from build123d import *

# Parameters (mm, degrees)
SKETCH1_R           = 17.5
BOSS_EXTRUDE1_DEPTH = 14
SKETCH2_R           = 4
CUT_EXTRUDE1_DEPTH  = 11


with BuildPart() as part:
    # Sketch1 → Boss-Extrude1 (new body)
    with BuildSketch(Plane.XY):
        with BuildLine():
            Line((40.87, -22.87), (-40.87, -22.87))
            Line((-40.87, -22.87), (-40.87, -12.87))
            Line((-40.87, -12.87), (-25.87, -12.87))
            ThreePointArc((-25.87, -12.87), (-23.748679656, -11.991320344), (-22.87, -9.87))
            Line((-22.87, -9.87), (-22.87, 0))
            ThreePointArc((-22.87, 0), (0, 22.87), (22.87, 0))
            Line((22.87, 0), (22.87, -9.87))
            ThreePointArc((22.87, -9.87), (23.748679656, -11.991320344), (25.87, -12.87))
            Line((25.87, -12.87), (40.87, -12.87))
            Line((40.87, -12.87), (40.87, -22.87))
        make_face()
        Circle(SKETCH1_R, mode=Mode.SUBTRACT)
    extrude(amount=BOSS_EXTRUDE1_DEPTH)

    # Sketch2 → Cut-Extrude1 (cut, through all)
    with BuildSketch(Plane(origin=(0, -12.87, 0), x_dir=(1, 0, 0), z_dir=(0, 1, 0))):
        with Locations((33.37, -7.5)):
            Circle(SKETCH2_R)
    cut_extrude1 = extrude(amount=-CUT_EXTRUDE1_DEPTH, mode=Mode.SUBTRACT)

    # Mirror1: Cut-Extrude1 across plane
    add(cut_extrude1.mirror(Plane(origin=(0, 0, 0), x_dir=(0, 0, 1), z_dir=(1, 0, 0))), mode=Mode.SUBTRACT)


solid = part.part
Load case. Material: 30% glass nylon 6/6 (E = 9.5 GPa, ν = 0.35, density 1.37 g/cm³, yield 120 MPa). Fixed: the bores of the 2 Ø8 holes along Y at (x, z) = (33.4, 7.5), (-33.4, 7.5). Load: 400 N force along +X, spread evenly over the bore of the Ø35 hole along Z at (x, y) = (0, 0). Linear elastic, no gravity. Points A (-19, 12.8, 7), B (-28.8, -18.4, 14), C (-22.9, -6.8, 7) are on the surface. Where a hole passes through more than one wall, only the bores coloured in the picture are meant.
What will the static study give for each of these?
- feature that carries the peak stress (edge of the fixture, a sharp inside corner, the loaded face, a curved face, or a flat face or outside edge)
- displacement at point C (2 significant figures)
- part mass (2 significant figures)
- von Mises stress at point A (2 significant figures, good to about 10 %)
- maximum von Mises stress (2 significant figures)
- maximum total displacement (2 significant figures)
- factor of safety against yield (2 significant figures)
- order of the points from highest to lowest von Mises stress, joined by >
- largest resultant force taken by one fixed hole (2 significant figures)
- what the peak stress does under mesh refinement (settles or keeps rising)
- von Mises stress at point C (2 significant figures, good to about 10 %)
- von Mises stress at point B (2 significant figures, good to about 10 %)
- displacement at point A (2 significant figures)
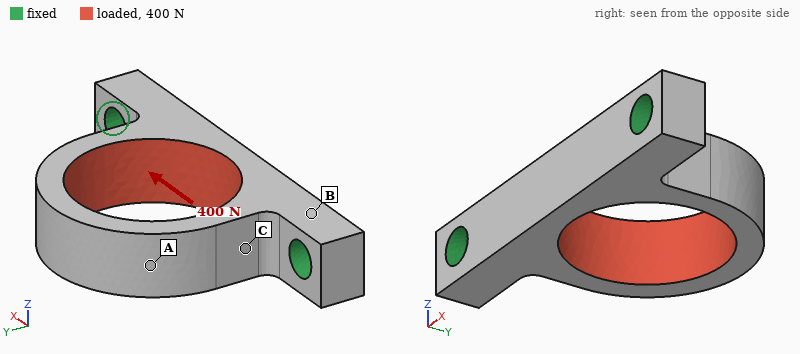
a curved face
17 µm
23 g
5.9 MPa
14 MPa
94 µm
8.5
C > A > B
230 N
settles
9.5 MPa
2.0 MPa
87 µm
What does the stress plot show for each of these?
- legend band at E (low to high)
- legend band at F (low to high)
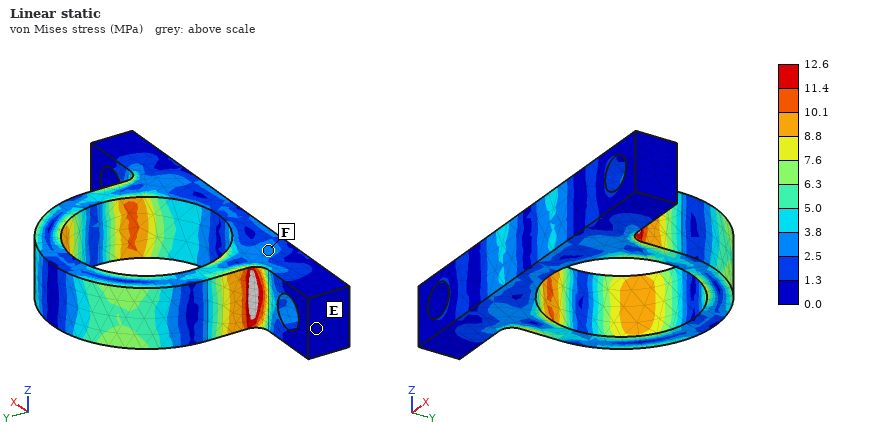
0.0 to 1.3 MPa
2.5 to 3.8 MPa
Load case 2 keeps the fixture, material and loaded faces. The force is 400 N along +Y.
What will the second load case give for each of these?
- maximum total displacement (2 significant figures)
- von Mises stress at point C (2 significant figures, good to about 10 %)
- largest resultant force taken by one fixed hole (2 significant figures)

24 µm
4.8 MPa
200 N
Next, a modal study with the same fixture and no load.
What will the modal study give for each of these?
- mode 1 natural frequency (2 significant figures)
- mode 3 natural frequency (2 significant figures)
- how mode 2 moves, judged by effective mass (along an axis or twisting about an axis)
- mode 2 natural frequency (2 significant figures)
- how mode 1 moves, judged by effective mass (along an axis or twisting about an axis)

2100 Hz
4700 Hz
along X
3100 Hz
along Z
